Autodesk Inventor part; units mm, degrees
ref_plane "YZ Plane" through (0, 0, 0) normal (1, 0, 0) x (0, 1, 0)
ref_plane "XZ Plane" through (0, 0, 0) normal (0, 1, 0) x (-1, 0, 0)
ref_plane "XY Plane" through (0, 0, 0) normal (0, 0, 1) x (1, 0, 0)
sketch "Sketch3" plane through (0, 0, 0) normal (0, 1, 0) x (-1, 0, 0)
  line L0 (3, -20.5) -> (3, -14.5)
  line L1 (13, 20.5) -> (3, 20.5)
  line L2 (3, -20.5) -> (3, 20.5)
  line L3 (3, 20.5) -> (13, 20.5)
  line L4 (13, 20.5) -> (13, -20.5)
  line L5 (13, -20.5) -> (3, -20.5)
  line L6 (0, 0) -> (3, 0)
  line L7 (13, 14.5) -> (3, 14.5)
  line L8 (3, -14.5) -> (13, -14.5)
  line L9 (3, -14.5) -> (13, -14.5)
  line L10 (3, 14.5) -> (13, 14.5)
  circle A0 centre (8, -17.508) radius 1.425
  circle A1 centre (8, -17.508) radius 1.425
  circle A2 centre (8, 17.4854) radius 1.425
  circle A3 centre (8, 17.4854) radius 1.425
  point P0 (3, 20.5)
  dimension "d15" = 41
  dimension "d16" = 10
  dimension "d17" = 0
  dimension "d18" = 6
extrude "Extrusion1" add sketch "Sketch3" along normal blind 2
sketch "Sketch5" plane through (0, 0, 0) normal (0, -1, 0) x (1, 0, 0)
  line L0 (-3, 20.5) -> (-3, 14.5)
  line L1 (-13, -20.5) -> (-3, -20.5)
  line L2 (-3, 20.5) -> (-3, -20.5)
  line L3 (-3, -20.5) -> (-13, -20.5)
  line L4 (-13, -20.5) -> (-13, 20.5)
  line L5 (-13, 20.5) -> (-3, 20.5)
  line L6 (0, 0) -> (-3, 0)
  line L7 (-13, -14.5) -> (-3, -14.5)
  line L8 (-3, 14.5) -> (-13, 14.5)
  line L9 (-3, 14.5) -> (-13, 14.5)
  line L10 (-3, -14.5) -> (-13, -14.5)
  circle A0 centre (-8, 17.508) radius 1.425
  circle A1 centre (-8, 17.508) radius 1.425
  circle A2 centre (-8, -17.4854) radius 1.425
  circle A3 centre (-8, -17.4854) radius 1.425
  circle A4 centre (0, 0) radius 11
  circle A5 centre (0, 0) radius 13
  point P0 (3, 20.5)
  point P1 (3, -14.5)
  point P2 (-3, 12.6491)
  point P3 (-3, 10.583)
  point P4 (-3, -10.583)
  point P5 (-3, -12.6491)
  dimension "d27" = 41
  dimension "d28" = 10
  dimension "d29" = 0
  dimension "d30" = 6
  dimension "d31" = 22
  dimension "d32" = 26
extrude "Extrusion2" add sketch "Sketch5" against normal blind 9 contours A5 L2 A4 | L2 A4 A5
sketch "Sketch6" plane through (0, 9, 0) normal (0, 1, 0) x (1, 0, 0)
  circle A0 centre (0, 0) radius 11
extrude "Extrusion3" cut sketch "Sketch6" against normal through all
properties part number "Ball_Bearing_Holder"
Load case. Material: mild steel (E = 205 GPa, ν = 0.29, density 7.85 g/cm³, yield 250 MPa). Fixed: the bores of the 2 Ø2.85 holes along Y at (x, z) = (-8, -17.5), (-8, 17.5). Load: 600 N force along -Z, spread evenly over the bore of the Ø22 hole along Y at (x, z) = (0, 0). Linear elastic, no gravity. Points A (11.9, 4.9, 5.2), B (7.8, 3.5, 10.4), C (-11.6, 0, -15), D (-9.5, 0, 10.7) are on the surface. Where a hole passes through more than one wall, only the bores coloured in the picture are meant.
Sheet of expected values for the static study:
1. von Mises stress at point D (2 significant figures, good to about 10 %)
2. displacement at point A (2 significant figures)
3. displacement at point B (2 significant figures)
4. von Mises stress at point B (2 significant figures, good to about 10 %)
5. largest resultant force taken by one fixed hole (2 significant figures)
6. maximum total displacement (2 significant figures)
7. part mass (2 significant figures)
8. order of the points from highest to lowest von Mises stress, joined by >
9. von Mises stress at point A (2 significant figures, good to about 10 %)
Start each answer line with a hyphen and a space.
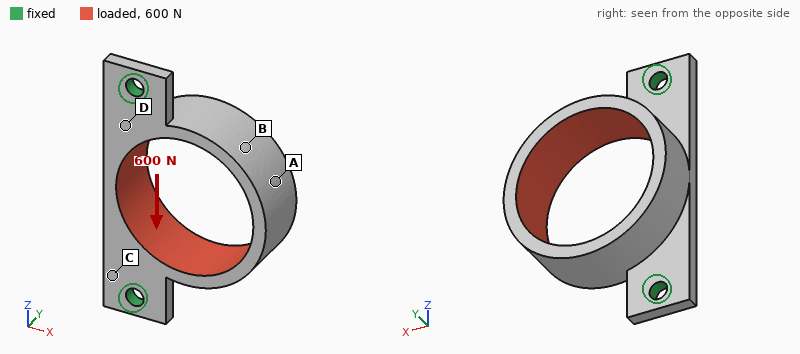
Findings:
- 23 MPa
- 33 µm
- 33 µm
- 63 MPa
- 330 N
- 37 µm
- 14 g
- B > A > D > C
- 48 MPa
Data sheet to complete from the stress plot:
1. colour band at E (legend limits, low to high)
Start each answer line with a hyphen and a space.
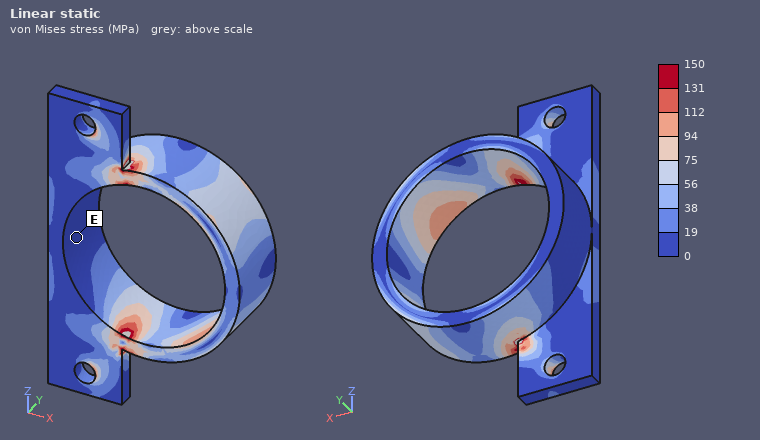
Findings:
- 0 to 19 MPa
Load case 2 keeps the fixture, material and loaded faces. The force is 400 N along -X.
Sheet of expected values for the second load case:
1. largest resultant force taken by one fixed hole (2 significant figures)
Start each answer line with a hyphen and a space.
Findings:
- 210 N
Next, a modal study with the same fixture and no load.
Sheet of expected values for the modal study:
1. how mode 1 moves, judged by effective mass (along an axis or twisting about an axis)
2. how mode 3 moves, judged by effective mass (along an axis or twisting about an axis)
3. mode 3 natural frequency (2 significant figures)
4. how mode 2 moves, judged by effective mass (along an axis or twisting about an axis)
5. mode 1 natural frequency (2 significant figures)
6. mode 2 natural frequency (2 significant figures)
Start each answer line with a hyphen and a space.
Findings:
- along Y
- along Y
- 10 kHz
- along Z
- 3000 Hz
- 6900 Hz
